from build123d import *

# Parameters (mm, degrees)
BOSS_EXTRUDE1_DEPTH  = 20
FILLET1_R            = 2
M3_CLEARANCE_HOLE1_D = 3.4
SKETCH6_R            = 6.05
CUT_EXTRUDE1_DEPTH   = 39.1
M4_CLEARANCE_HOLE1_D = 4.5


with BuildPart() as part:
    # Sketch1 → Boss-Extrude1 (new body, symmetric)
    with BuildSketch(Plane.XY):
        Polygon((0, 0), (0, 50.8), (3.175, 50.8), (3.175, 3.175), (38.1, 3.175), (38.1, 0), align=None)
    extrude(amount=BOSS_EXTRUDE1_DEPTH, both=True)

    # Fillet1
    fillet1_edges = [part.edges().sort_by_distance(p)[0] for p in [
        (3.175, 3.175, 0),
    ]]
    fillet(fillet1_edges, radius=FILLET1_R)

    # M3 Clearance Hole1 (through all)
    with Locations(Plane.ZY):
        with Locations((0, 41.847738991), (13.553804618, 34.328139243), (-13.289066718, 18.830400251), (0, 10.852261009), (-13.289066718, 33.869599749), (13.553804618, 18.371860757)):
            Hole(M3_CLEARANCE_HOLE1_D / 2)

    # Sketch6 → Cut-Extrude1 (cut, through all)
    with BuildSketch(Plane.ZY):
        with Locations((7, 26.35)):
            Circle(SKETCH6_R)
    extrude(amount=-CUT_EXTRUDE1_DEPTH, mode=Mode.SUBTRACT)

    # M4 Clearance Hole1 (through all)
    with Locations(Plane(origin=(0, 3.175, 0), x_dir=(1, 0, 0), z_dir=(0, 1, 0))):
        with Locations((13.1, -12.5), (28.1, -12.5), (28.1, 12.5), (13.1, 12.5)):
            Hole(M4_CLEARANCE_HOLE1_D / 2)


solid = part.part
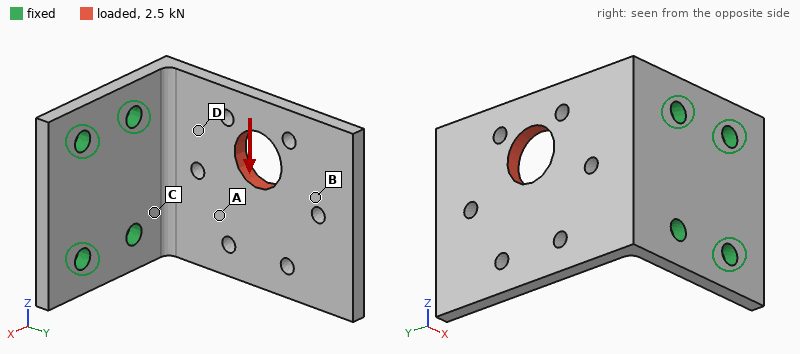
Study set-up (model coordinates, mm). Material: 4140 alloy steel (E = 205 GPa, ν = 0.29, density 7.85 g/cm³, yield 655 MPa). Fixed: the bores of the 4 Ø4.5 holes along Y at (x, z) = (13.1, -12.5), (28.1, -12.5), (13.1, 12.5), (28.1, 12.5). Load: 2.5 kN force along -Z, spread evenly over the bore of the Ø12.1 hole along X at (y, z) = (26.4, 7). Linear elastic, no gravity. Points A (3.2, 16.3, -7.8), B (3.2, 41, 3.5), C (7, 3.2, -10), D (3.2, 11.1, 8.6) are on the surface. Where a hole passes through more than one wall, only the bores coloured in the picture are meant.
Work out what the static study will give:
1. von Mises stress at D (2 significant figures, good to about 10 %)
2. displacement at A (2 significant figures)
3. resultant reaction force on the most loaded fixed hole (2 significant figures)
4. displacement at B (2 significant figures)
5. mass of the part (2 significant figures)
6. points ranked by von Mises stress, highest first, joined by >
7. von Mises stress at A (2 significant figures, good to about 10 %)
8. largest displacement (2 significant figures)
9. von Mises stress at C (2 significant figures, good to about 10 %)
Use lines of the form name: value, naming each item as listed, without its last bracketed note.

von Mises stress at D: 150 MPa
displacement at A: 0.082 mm
resultant reaction force on the most loaded fixed hole: 2.8 kN
displacement at B: 0.18 mm
mass of the part: 80 g
points ranked by von Mises stress, highest first, joined by >: C > D > A > B
von Mises stress at A: 93 MPa
largest displacement: 0.26 mm
von Mises stress at C: 270 MPa
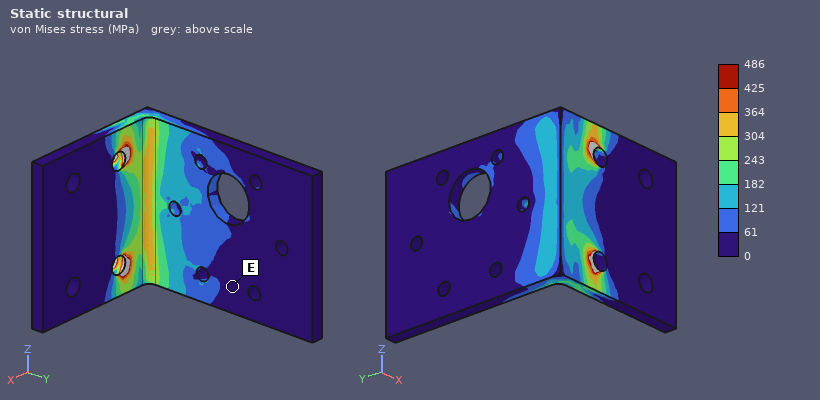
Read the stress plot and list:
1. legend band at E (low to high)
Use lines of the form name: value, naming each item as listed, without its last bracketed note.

legend band at E: 0 to 61 MPa
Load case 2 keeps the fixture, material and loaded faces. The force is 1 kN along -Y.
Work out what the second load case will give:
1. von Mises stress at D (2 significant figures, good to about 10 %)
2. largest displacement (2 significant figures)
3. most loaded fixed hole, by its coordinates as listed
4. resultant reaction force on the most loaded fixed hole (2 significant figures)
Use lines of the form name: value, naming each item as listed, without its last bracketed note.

von Mises stress at D: 21 MPa
largest displacement: 0.15 mm
most loaded fixed hole, by its coordinates as listed: (13.1, 12.5)
resultant reaction force on the most loaded fixed hole: 840 N
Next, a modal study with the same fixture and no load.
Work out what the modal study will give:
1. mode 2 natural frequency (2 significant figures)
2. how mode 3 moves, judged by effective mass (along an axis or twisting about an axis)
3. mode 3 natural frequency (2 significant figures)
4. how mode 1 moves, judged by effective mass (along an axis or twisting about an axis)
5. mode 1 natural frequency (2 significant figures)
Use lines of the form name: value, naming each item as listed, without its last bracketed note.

mode 2 natural frequency: 2400 Hz
how mode 3 moves, judged by effective mass: along Z
mode 3 natural frequency: 3300 Hz
how mode 1 moves, judged by effective mass: along X
mode 1 natural frequency: 840 Hz
